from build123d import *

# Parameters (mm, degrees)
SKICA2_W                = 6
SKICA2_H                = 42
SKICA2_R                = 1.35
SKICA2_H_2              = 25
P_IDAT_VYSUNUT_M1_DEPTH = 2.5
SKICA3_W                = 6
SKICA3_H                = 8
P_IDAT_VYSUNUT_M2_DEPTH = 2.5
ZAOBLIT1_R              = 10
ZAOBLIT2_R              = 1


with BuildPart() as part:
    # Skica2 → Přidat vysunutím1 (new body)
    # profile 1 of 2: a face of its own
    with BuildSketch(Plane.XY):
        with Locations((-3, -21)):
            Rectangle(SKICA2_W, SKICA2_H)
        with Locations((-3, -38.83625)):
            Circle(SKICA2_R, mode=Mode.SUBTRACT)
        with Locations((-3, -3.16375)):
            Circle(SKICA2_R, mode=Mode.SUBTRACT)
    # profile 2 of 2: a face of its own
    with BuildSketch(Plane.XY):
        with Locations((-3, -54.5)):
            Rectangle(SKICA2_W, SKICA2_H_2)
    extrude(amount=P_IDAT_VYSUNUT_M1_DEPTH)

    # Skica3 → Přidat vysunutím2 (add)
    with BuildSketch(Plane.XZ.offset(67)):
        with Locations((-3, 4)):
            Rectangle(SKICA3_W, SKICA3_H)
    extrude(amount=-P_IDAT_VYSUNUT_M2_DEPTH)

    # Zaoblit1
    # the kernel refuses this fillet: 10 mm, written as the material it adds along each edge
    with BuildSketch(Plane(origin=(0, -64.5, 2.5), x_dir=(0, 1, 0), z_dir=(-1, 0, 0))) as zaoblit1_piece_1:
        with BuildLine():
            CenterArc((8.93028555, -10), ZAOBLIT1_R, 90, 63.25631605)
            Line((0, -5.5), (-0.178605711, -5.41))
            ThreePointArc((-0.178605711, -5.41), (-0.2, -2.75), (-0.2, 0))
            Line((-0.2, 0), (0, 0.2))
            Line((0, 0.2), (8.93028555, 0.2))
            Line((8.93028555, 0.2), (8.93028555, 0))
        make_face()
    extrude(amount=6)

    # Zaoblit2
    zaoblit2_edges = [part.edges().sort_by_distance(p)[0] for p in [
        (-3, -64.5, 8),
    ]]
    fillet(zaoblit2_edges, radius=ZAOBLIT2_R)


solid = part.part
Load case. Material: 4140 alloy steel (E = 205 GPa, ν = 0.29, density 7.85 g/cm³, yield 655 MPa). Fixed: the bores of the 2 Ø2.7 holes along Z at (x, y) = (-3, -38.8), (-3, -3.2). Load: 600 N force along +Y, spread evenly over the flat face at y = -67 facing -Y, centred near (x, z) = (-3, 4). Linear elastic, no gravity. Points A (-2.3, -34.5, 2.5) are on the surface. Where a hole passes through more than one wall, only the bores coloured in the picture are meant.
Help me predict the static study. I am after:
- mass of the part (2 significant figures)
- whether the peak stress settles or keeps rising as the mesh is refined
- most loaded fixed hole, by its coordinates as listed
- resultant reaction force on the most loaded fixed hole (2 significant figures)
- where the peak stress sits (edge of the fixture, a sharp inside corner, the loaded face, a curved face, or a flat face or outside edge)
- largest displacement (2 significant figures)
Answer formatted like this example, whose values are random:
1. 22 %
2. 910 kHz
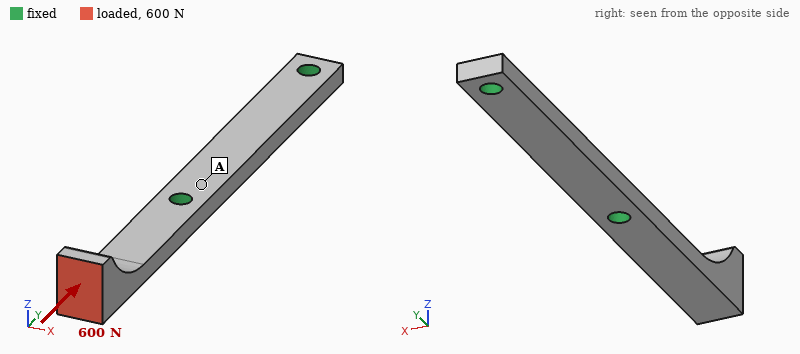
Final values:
1. 9.0 g
2. keeps rising
3. (-3, -38.8)
4. 590 N
5. edge of the fixture
6. 0.38 mm
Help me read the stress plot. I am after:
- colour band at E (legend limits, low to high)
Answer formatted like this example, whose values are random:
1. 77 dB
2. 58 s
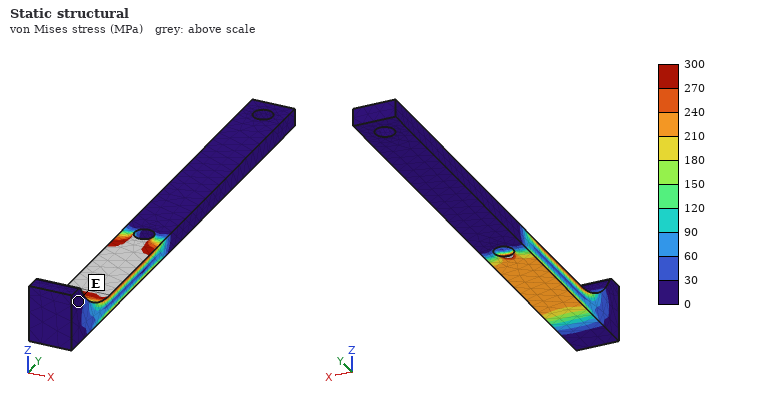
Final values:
1. 0 to 30 MPa
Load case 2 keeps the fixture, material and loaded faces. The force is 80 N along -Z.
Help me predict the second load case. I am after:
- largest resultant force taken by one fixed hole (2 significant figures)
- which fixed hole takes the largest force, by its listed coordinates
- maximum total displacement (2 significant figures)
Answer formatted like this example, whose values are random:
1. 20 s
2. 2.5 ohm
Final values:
1. 80 N
2. (-3, -38.8)
3. 0.35 mm
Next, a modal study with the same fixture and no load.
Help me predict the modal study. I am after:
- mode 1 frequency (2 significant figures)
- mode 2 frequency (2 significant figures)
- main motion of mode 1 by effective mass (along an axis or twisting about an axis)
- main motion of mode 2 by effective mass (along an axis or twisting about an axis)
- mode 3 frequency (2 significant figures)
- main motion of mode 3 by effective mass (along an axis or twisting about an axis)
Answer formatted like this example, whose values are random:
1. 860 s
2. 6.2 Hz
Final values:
1. 1800 Hz
2. 3800 Hz
3. along Z
4. along X
5. 11 kHz
6. along Z
